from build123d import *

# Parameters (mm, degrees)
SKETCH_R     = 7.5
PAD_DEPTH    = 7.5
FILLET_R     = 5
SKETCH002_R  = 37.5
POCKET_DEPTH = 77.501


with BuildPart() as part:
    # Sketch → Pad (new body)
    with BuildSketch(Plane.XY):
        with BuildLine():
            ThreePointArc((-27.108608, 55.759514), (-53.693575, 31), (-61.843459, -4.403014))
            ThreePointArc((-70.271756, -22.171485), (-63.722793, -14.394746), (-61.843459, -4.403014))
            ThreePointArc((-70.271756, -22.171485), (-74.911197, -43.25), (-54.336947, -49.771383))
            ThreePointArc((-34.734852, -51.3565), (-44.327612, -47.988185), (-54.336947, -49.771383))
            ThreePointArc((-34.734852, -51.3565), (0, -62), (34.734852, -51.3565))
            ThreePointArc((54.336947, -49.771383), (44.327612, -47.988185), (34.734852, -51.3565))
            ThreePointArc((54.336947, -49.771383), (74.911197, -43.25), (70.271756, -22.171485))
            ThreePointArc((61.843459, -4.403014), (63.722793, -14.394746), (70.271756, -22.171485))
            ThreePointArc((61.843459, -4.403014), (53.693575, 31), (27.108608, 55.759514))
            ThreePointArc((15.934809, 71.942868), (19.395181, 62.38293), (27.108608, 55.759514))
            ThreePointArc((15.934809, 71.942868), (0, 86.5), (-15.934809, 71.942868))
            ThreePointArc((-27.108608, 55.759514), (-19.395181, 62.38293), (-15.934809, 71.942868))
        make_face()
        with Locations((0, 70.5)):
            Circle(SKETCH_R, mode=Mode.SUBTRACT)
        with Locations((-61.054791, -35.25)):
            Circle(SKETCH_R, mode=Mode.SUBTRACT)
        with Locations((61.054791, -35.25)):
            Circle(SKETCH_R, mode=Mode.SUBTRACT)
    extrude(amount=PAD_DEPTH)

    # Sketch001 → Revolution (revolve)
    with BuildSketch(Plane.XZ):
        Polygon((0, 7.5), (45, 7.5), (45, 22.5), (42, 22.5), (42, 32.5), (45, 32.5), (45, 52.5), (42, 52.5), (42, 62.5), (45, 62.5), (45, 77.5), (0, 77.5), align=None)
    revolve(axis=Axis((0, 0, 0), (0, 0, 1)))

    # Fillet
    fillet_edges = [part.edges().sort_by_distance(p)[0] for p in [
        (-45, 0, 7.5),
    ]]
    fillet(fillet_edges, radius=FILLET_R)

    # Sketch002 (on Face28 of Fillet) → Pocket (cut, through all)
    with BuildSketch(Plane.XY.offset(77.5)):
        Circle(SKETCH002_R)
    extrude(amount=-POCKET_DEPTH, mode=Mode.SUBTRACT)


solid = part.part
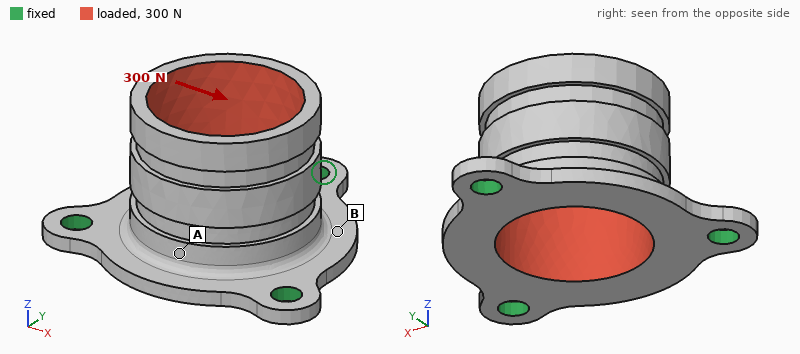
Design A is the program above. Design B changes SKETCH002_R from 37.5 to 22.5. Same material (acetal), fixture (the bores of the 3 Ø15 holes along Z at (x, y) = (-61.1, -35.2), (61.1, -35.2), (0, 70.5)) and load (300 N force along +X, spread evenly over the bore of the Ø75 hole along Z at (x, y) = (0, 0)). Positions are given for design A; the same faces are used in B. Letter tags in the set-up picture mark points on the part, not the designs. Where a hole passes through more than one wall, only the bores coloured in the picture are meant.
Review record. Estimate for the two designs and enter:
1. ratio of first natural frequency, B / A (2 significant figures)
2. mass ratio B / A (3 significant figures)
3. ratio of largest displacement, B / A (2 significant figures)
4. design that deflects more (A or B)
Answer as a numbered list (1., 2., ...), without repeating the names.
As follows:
1. 0.87
2. 2.14
3. 0.55
4. A
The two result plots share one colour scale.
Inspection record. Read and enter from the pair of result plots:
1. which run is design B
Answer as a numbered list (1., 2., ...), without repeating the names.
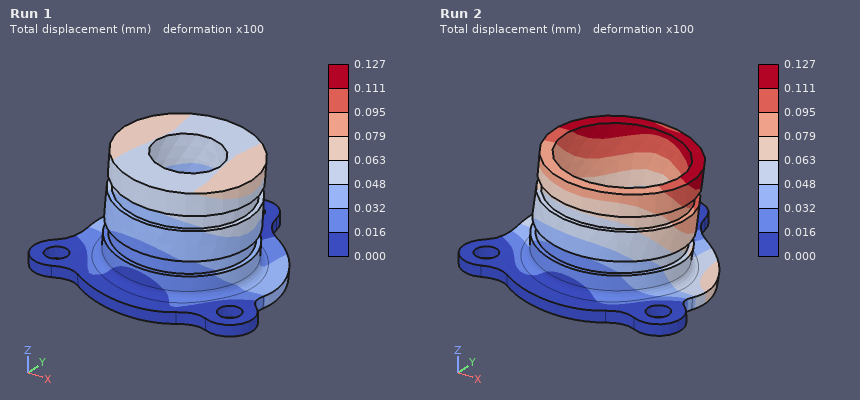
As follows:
1. Run 1
